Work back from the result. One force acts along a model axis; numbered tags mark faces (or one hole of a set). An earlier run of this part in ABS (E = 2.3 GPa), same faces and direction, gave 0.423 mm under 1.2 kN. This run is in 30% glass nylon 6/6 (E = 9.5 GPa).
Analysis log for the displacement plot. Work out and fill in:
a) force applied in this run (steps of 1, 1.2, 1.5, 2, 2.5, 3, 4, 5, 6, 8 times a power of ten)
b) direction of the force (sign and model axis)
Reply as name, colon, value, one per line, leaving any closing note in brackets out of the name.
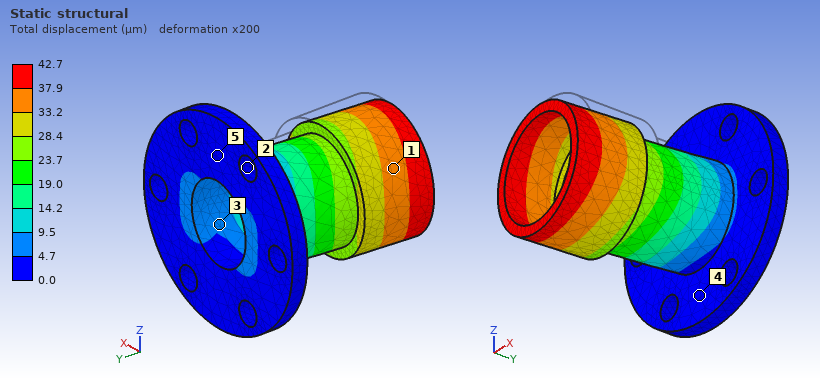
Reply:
force applied in this run: 500 N
direction of the force: -X
